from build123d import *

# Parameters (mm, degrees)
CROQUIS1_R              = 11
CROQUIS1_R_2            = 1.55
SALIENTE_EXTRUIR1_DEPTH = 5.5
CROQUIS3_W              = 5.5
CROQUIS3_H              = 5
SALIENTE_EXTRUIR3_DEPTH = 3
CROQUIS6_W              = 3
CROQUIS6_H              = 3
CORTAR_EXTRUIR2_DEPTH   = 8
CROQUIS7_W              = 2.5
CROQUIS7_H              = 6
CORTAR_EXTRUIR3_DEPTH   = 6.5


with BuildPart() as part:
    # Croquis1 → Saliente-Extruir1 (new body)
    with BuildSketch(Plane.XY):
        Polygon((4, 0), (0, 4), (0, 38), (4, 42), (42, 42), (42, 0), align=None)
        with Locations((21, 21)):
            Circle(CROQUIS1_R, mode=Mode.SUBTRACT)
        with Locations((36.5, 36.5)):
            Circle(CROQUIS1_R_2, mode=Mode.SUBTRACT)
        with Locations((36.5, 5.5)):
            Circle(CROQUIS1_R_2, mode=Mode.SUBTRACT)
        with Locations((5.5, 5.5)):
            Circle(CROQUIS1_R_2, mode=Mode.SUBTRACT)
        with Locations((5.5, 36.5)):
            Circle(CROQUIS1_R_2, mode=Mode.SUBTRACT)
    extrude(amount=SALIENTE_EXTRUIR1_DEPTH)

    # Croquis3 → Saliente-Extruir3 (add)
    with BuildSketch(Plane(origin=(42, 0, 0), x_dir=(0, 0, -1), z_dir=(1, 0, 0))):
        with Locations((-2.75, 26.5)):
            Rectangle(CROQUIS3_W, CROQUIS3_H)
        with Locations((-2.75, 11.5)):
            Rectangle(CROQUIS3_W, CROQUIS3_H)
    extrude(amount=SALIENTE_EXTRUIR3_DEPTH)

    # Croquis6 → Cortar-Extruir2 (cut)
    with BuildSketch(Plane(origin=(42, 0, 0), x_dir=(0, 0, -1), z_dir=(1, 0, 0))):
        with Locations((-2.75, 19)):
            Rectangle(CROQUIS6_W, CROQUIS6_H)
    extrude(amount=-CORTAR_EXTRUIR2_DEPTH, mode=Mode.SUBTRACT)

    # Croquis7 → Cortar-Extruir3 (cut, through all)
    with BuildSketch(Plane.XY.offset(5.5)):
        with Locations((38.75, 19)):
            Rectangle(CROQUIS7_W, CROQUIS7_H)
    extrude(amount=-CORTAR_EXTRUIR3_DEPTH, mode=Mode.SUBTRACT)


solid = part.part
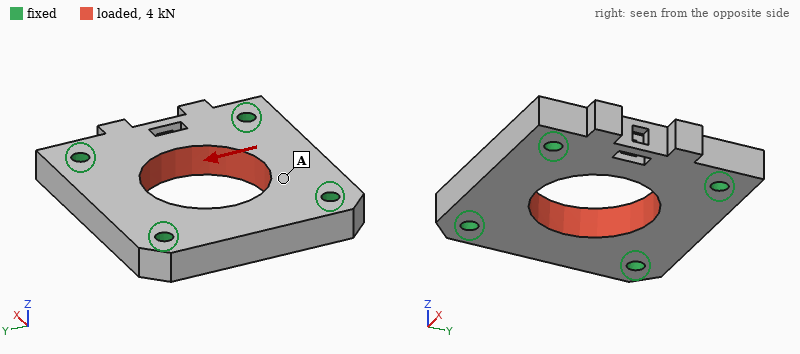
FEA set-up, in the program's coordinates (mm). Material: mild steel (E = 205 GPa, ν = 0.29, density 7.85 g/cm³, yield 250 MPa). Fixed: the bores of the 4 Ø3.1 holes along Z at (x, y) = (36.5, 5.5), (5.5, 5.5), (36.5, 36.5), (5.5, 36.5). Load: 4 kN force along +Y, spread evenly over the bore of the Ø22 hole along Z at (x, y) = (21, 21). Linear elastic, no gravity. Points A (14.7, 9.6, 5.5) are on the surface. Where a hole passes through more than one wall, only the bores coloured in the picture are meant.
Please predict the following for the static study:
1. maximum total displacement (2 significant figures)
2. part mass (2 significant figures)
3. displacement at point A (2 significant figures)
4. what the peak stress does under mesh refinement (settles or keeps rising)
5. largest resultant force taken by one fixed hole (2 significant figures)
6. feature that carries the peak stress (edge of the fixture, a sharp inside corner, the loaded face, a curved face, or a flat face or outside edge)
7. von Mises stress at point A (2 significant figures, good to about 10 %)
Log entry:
2.4 µm
58 g
1.6 µm
keeps rising
1.1 kN
edge of the fixture
14 MPa
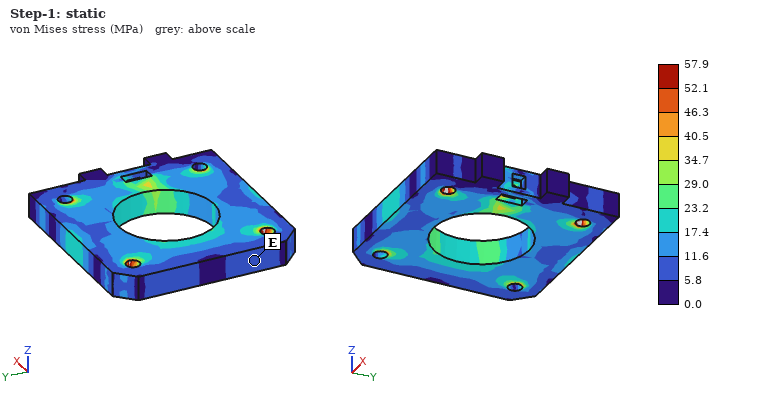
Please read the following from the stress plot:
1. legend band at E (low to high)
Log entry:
5.8 to 11.6 MPa
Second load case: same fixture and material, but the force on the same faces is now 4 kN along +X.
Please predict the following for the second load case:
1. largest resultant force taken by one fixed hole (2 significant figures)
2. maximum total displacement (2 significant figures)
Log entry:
1.1 kN
2.7 µm
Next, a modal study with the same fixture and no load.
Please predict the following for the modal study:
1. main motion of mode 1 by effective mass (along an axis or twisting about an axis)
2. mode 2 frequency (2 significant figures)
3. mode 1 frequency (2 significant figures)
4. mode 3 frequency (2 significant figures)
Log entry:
along Z
25 kHz
24 kHz
26 kHz
